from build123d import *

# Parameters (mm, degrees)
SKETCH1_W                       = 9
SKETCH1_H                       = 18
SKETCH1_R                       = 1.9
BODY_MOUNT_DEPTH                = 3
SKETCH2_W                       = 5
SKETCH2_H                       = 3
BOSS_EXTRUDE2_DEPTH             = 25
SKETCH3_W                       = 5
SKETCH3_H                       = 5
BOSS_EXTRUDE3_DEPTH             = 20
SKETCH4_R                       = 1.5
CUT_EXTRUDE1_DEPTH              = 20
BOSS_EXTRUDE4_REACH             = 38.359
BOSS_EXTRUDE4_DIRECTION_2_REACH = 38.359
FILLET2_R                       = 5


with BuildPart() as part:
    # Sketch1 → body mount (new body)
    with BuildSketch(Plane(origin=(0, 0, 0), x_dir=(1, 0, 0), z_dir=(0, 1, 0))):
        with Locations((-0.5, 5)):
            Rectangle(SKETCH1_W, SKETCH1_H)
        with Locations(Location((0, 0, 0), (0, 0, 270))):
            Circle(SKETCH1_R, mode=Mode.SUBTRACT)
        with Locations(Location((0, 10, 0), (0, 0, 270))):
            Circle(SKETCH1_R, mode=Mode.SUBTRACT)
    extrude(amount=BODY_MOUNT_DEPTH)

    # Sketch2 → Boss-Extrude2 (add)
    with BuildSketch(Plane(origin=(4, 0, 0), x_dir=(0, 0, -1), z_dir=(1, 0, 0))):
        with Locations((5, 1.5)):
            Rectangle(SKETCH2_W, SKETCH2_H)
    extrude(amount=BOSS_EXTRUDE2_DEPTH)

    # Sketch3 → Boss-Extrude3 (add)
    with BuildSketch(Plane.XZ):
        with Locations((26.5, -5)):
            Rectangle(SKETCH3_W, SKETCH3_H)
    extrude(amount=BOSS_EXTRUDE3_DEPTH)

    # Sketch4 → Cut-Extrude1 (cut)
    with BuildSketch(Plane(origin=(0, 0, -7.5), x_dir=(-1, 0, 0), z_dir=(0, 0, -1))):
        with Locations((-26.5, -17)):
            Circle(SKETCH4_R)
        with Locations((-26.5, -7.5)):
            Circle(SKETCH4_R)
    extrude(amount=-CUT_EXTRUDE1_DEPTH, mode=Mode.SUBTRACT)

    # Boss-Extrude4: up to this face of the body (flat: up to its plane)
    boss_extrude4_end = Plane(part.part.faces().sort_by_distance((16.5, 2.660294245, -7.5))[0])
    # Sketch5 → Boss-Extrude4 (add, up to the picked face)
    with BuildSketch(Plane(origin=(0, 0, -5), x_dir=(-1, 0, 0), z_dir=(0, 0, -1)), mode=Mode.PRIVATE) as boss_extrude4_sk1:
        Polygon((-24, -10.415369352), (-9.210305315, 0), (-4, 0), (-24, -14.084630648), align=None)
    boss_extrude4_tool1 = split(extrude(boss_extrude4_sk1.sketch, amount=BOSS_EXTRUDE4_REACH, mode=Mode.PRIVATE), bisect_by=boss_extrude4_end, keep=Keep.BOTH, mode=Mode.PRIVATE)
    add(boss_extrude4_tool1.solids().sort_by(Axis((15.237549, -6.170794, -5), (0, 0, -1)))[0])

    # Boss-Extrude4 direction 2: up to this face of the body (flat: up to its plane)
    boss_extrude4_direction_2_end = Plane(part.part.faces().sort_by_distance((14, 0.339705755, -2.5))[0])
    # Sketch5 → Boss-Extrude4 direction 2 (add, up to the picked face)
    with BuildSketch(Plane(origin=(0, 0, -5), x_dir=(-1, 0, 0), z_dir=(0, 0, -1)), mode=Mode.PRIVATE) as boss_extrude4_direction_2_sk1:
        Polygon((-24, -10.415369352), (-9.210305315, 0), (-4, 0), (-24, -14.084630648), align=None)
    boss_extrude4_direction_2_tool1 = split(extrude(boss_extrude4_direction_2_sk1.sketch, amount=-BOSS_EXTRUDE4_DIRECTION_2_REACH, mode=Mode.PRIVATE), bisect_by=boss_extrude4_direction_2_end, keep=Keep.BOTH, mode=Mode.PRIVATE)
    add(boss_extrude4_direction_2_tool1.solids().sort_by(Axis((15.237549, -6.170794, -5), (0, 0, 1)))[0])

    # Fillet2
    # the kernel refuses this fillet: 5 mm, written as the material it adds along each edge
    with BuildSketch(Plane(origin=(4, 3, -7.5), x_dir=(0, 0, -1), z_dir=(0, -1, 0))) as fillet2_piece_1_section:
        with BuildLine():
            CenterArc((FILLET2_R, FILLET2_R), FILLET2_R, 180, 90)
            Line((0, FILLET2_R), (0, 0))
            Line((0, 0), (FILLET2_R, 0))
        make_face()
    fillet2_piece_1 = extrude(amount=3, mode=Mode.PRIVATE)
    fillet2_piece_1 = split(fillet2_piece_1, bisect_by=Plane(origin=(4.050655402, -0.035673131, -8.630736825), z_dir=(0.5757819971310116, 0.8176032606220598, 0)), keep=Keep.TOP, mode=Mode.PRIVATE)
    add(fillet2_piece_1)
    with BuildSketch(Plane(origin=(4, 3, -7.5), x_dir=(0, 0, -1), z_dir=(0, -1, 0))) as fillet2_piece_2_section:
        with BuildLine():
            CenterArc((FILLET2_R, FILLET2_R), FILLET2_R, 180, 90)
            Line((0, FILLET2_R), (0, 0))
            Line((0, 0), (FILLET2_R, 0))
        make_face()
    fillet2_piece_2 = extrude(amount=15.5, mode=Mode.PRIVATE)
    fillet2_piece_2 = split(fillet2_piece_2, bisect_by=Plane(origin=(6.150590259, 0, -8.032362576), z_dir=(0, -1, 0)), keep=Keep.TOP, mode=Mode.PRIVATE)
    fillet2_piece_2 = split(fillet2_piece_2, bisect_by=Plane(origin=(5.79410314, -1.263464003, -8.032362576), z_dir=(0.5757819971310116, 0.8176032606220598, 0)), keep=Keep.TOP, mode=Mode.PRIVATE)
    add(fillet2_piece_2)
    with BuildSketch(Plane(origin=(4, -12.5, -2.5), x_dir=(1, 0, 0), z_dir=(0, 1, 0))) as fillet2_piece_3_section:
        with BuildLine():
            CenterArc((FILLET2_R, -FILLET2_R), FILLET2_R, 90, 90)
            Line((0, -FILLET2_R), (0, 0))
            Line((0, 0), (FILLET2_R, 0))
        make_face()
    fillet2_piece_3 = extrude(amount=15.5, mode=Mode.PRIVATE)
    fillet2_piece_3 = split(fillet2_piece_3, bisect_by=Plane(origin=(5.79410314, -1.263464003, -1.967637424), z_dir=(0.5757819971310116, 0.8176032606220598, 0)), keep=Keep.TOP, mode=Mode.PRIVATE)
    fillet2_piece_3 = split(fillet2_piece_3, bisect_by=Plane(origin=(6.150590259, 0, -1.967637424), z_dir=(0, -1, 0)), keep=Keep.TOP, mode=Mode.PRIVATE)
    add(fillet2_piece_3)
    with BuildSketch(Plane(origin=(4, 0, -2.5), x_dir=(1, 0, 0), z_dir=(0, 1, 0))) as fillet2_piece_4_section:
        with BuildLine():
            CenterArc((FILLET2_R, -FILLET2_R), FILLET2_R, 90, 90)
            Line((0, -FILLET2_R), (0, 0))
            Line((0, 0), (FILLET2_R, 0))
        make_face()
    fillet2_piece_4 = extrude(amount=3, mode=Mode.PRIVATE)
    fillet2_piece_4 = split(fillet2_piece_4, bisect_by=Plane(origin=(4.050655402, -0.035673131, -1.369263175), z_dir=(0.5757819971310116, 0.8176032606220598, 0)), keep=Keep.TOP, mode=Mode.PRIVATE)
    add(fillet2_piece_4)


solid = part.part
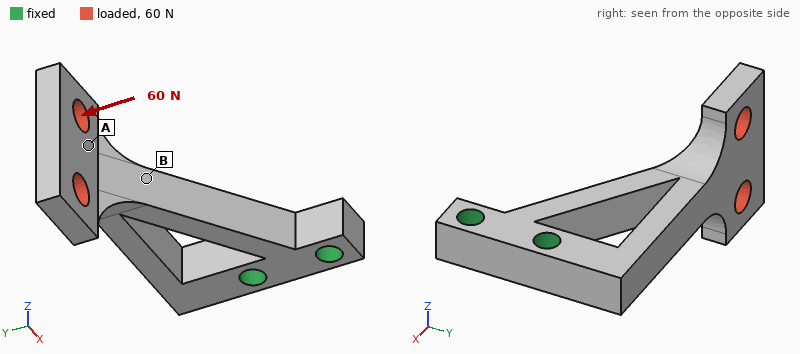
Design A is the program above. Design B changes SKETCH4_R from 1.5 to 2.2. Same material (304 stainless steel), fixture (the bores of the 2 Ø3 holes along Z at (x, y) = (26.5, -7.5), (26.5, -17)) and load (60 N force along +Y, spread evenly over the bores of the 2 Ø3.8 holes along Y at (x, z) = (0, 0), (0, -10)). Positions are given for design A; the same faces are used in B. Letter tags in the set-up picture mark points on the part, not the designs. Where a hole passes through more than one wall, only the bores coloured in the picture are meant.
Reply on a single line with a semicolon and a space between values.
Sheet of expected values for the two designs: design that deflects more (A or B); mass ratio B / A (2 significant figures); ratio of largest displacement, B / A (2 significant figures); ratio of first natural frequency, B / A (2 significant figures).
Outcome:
A; 0.95; 0.88; 1.0
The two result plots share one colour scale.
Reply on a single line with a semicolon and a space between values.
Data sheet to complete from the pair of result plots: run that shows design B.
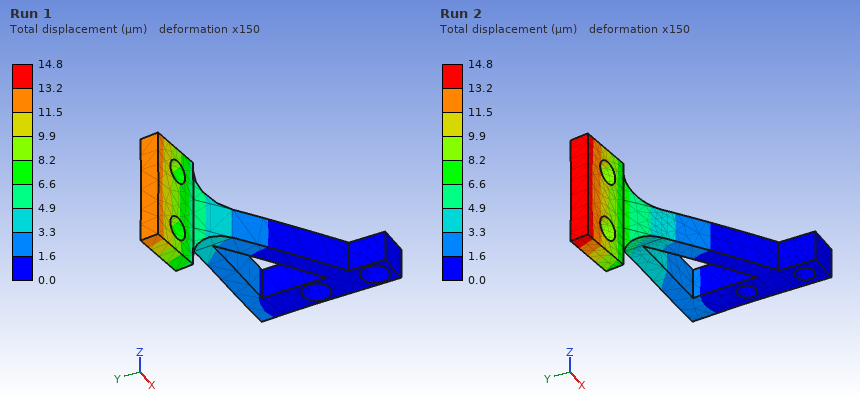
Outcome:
Run 1
